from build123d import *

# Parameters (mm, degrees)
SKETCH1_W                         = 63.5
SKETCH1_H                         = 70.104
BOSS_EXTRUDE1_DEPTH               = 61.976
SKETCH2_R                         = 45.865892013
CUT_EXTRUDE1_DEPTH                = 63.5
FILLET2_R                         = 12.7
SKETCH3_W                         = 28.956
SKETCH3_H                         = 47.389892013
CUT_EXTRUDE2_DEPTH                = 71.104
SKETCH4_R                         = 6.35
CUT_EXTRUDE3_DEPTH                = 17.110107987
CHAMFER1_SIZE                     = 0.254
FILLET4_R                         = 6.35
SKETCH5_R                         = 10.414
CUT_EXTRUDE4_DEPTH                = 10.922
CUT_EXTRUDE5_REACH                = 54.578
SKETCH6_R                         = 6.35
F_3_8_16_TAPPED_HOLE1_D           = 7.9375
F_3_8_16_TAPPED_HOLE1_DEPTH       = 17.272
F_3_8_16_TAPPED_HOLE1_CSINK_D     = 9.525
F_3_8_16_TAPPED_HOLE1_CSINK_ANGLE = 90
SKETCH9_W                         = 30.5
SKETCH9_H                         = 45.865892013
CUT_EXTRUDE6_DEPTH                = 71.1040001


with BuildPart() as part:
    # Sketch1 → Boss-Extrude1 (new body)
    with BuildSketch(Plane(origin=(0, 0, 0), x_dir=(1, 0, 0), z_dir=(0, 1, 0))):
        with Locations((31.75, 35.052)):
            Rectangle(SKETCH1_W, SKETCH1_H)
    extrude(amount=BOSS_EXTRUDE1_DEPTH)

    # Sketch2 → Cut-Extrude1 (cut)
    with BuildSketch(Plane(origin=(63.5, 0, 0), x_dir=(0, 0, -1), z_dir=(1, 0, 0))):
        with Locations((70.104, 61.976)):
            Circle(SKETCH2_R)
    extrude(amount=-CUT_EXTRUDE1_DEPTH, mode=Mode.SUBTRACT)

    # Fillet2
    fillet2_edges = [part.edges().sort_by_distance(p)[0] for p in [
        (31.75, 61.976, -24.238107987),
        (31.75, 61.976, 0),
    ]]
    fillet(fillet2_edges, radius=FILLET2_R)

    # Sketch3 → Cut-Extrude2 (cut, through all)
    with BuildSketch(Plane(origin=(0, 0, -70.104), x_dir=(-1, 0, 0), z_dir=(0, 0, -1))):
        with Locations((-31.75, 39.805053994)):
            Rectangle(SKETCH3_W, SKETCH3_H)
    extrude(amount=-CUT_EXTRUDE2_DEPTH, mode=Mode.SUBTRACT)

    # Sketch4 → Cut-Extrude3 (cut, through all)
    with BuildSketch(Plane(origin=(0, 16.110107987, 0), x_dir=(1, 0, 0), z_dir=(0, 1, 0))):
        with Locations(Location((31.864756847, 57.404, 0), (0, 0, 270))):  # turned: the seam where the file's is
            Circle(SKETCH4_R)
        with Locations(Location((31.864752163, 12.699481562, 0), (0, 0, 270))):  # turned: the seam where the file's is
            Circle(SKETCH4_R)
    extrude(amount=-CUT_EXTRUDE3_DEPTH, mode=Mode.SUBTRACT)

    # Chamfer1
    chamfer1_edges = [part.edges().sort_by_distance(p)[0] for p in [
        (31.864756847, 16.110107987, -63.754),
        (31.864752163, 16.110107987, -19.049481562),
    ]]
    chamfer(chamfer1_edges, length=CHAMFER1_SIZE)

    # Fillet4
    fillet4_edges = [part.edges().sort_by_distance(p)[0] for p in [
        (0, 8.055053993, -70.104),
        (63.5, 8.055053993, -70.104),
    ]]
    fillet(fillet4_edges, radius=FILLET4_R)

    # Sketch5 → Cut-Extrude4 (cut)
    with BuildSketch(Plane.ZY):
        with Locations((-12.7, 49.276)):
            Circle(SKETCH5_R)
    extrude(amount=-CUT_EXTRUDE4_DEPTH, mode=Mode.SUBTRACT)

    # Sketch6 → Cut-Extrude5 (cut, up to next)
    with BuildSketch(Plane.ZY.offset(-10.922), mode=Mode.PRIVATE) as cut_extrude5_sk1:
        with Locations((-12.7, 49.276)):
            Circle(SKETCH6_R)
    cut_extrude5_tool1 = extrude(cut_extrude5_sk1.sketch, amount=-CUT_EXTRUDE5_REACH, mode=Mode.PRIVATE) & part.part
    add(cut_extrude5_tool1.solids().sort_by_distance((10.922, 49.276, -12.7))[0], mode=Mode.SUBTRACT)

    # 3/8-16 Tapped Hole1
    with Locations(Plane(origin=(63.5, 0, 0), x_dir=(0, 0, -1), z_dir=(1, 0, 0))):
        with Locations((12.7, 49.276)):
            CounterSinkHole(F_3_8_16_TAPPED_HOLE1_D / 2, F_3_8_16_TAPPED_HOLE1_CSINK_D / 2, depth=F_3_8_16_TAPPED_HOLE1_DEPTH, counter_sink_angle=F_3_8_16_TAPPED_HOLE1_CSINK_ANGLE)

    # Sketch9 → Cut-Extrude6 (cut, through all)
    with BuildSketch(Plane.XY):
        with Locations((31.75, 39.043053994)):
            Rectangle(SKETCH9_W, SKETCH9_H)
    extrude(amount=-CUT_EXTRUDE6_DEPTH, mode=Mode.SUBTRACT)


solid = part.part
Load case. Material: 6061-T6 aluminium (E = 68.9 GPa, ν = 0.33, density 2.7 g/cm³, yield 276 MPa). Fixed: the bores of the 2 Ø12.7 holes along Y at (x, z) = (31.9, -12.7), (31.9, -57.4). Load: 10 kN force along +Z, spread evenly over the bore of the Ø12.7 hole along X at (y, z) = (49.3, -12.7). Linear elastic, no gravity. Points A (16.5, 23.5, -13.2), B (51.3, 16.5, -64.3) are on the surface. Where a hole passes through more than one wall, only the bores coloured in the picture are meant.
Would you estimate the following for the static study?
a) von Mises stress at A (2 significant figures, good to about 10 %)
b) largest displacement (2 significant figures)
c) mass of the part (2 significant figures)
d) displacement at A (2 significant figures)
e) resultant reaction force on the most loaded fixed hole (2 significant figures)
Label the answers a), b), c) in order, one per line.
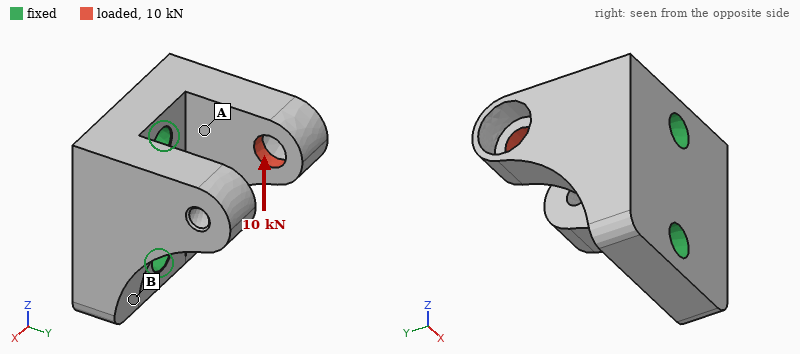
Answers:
a) 61 MPa
b) 0.25 mm
c) 300 g
d) 0.049 mm
e) 9.8 kN
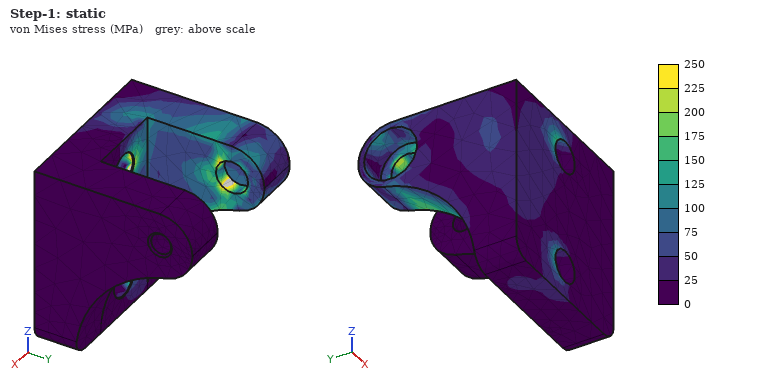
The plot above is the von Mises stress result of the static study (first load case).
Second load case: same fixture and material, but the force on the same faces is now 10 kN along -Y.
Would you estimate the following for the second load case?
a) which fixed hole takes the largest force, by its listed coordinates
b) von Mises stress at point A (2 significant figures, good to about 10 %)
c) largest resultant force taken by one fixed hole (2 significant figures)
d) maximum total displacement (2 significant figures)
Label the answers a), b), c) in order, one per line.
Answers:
a) (31.9, -12.7)
b) 58 MPa
c) 9.3 kN
d) 94 µm
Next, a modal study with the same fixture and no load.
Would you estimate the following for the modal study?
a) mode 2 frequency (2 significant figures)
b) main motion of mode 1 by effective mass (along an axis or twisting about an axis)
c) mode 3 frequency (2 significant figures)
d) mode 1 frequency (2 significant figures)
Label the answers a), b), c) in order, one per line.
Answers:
a) 5000 Hz
b) along X
c) 7700 Hz
d) 4200 Hz
